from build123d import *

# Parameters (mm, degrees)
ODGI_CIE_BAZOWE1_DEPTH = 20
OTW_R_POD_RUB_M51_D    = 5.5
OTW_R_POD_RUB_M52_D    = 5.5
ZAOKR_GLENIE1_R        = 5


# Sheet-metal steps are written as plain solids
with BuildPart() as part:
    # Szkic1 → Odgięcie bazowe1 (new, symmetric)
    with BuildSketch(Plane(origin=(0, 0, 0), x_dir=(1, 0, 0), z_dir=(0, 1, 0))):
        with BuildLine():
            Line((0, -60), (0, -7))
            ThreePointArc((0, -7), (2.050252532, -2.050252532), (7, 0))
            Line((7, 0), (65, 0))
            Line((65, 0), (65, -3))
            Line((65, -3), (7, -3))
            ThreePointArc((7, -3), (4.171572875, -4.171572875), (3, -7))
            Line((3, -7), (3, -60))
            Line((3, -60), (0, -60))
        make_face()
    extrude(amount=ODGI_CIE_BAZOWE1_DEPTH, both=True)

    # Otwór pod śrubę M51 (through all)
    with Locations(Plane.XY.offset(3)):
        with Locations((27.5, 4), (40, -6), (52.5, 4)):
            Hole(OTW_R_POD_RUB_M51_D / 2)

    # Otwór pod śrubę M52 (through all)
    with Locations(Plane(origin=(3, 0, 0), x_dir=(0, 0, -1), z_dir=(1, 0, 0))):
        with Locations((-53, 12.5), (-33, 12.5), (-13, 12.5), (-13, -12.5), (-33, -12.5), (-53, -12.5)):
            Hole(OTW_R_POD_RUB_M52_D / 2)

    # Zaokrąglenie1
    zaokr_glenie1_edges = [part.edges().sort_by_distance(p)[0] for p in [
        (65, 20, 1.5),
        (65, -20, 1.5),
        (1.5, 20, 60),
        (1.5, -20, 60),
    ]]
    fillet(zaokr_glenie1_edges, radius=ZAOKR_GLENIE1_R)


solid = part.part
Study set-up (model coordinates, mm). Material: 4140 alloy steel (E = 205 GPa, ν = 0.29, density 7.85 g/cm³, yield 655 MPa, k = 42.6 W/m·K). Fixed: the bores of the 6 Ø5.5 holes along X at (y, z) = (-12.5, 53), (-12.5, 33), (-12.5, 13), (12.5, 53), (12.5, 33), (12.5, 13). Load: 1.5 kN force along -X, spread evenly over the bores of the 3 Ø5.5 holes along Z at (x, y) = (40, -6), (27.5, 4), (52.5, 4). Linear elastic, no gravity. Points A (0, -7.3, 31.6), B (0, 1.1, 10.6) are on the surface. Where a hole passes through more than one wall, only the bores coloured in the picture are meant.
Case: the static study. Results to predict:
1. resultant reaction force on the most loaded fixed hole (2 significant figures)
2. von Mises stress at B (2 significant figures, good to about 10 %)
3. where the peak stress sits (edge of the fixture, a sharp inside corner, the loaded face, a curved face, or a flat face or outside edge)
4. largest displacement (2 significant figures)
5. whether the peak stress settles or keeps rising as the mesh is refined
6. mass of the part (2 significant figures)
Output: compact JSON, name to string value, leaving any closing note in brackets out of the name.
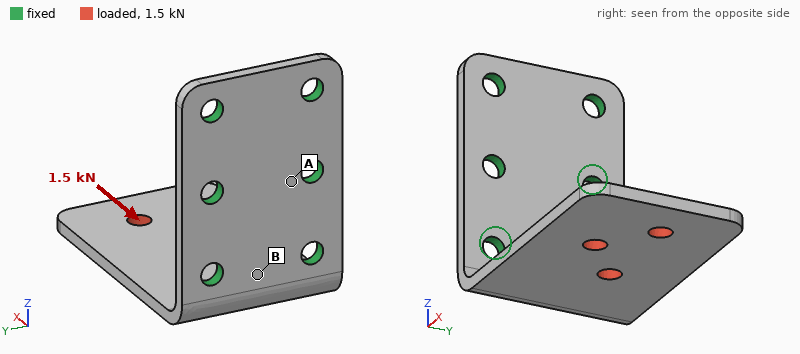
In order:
{"resultant reaction force on the most loaded fixed hole": "840 N", "von Mises stress at B": "88 MPa", "where the peak stress sits": "edge of the fixture", "largest displacement": "0.28 mm", "whether the peak stress settles or keeps rising as the mesh is refined": "keeps rising", "mass of the part": "110 g"}
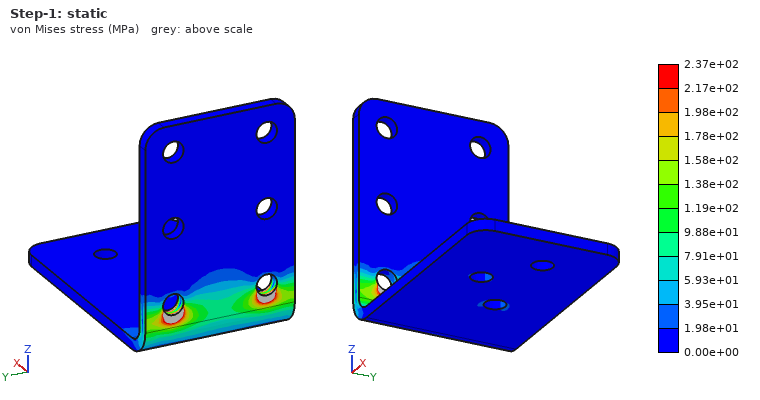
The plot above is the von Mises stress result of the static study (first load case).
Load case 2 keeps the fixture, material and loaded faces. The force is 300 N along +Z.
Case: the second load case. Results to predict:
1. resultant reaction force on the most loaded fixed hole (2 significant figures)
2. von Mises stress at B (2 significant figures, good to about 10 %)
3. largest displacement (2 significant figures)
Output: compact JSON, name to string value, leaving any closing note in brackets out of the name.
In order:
{"resultant reaction force on the most loaded fixed hole": "140 N", "von Mises stress at B": "100 MPa", "largest displacement": "0.92 mm"}
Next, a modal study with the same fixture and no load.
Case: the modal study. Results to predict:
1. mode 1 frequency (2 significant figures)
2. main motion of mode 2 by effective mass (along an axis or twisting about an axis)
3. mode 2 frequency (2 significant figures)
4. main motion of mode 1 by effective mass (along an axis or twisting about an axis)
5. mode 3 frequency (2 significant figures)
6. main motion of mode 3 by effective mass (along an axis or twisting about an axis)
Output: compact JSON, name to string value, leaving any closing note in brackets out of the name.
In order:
{"mode 1 frequency": "520 Hz", "main motion of mode 2 by effective mass": "along Y", "mode 2 frequency": "1800 Hz", "main motion of mode 1 by effective mass": "along Z", "mode 3 frequency": "2500 Hz", "main motion of mode 3 by effective mass": "along Y"}
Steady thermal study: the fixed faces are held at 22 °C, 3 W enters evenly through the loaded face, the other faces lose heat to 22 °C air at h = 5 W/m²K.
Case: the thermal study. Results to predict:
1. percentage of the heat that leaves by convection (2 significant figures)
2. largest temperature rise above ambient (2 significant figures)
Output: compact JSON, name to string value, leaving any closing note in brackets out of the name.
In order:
{"percentage of the heat that leaves by convection": "16 %", "largest temperature rise above ambient": "26 K"}
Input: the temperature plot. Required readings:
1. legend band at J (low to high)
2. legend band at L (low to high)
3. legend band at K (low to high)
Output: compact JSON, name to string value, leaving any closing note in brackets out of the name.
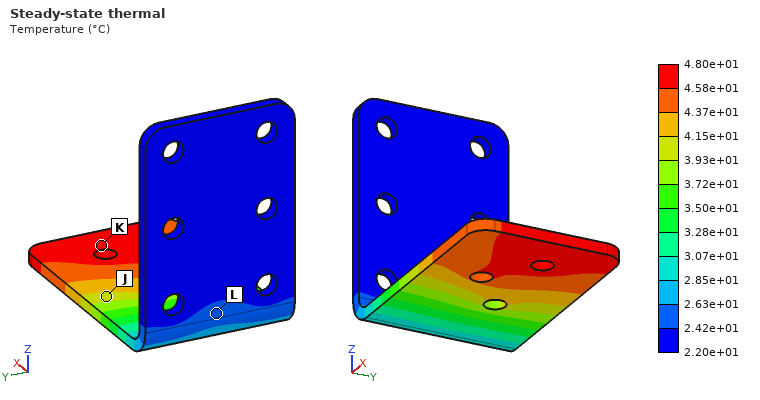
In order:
{"legend band at J": "3.93e+01 to 4.15e+01 °C", "legend band at L": "2.42e+01 to 2.63e+01 °C", "legend band at K": "4.58e+01 to 4.80e+01 °C"}
